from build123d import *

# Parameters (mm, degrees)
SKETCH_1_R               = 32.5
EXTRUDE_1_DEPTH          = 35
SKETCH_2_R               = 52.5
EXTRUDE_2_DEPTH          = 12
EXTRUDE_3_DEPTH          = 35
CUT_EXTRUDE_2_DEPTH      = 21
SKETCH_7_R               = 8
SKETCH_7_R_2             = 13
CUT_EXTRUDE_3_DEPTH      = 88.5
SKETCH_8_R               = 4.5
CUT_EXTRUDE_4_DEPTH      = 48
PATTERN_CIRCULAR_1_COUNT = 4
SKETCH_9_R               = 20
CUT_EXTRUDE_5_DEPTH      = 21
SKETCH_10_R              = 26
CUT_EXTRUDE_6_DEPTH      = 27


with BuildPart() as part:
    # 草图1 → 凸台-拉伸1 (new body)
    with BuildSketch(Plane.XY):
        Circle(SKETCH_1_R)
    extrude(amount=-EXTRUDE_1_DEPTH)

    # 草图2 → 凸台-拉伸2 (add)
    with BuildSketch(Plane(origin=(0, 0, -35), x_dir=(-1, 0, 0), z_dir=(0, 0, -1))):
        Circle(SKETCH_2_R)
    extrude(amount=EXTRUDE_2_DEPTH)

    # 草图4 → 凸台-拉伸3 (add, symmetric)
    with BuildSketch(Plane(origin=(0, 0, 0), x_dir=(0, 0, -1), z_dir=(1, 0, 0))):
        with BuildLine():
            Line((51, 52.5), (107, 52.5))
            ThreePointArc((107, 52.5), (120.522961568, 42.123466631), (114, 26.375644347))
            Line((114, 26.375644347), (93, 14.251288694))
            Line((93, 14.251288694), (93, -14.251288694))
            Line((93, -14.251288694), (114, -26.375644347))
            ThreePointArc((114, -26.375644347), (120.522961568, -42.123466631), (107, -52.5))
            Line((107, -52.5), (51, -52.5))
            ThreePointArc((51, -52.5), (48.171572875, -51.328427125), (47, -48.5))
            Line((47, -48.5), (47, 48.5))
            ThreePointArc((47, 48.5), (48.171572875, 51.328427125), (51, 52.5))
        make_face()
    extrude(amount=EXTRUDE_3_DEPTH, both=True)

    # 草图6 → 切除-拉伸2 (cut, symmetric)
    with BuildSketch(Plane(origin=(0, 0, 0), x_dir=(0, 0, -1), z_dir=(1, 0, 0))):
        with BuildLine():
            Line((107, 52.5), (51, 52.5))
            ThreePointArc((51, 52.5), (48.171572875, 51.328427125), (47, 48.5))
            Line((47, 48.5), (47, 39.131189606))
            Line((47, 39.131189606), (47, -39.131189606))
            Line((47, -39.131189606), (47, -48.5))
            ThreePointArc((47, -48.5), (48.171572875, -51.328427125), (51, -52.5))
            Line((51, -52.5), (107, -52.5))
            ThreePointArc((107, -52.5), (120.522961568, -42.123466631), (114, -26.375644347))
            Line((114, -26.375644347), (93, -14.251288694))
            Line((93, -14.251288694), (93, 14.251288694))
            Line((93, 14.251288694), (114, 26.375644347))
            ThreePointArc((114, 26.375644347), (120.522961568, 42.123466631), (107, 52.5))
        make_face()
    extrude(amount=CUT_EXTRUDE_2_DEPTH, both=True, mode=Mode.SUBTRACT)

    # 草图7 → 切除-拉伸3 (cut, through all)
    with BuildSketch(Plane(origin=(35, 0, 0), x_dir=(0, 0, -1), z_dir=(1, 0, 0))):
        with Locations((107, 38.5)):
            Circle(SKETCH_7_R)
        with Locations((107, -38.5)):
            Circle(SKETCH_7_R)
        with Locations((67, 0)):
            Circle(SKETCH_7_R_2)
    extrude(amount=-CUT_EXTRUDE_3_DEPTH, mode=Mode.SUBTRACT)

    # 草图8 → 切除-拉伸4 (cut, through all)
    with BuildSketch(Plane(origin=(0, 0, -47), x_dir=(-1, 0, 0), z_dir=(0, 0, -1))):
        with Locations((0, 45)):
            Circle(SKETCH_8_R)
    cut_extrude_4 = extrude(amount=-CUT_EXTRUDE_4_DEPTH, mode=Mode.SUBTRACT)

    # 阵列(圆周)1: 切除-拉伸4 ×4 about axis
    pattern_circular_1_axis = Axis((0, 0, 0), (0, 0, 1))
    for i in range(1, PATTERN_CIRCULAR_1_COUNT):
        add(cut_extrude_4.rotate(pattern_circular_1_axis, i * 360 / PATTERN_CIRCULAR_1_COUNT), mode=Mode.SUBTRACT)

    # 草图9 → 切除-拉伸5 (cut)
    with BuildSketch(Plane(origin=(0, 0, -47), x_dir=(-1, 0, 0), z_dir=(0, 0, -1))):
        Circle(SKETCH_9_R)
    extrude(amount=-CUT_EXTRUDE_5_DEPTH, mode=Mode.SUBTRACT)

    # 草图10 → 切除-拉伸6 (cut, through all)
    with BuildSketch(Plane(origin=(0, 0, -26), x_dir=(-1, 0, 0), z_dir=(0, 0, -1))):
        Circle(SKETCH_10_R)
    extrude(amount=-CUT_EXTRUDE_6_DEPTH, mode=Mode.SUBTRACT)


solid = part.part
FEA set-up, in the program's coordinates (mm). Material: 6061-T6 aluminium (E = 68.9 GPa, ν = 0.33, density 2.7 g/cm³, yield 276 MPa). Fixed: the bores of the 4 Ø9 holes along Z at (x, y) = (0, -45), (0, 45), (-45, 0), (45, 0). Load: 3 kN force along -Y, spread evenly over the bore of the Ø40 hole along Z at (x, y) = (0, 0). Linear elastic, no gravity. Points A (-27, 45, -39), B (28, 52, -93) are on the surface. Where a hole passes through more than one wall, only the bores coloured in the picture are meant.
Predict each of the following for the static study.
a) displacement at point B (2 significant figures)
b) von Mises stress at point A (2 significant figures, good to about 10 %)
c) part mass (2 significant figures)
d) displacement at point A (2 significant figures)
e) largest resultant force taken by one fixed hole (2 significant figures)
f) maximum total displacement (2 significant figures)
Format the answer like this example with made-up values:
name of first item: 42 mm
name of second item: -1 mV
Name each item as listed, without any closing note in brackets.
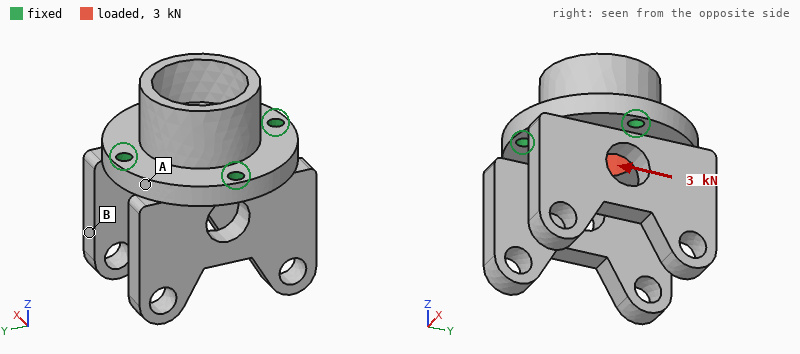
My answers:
displacement at point B: 0.76 µm
von Mises stress at point A: 1.0 MPa
part mass: 780 g
displacement at point A: 0.78 µm
largest resultant force taken by one fixed hole: 880 N
maximum total displacement: 1.4 µm
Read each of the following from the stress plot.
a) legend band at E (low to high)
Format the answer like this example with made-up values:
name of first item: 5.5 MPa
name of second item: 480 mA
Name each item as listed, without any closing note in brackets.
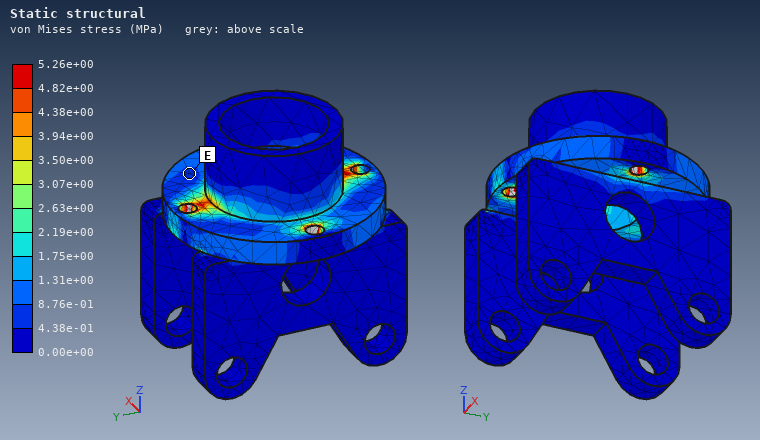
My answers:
legend band at E: 4.38e-01 to 8.76e-01 MPa
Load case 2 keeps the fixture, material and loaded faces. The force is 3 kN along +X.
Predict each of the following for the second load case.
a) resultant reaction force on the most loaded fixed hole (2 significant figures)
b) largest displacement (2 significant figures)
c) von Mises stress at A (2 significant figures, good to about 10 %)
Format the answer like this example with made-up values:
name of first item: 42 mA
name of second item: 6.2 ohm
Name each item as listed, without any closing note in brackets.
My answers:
resultant reaction force on the most loaded fixed hole: 900 N
largest displacement: 1.4 µm
von Mises stress at A: 0.93 MPa
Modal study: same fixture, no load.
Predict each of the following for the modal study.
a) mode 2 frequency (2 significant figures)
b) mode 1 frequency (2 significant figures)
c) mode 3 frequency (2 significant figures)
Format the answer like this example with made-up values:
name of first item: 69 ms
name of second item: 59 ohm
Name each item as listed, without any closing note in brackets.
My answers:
mode 2 frequency: 2100 Hz
mode 1 frequency: 2100 Hz
mode 3 frequency: 2600 Hz
